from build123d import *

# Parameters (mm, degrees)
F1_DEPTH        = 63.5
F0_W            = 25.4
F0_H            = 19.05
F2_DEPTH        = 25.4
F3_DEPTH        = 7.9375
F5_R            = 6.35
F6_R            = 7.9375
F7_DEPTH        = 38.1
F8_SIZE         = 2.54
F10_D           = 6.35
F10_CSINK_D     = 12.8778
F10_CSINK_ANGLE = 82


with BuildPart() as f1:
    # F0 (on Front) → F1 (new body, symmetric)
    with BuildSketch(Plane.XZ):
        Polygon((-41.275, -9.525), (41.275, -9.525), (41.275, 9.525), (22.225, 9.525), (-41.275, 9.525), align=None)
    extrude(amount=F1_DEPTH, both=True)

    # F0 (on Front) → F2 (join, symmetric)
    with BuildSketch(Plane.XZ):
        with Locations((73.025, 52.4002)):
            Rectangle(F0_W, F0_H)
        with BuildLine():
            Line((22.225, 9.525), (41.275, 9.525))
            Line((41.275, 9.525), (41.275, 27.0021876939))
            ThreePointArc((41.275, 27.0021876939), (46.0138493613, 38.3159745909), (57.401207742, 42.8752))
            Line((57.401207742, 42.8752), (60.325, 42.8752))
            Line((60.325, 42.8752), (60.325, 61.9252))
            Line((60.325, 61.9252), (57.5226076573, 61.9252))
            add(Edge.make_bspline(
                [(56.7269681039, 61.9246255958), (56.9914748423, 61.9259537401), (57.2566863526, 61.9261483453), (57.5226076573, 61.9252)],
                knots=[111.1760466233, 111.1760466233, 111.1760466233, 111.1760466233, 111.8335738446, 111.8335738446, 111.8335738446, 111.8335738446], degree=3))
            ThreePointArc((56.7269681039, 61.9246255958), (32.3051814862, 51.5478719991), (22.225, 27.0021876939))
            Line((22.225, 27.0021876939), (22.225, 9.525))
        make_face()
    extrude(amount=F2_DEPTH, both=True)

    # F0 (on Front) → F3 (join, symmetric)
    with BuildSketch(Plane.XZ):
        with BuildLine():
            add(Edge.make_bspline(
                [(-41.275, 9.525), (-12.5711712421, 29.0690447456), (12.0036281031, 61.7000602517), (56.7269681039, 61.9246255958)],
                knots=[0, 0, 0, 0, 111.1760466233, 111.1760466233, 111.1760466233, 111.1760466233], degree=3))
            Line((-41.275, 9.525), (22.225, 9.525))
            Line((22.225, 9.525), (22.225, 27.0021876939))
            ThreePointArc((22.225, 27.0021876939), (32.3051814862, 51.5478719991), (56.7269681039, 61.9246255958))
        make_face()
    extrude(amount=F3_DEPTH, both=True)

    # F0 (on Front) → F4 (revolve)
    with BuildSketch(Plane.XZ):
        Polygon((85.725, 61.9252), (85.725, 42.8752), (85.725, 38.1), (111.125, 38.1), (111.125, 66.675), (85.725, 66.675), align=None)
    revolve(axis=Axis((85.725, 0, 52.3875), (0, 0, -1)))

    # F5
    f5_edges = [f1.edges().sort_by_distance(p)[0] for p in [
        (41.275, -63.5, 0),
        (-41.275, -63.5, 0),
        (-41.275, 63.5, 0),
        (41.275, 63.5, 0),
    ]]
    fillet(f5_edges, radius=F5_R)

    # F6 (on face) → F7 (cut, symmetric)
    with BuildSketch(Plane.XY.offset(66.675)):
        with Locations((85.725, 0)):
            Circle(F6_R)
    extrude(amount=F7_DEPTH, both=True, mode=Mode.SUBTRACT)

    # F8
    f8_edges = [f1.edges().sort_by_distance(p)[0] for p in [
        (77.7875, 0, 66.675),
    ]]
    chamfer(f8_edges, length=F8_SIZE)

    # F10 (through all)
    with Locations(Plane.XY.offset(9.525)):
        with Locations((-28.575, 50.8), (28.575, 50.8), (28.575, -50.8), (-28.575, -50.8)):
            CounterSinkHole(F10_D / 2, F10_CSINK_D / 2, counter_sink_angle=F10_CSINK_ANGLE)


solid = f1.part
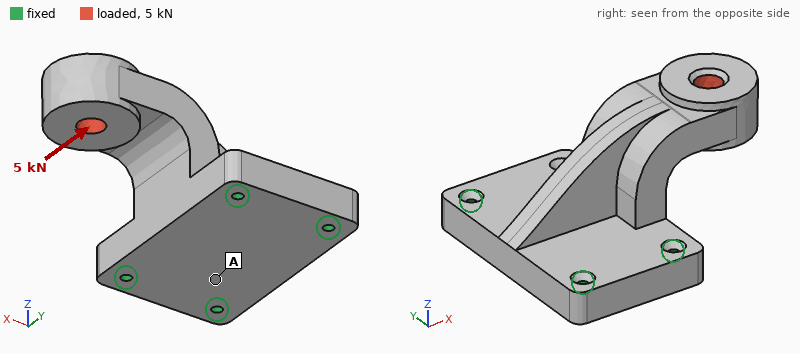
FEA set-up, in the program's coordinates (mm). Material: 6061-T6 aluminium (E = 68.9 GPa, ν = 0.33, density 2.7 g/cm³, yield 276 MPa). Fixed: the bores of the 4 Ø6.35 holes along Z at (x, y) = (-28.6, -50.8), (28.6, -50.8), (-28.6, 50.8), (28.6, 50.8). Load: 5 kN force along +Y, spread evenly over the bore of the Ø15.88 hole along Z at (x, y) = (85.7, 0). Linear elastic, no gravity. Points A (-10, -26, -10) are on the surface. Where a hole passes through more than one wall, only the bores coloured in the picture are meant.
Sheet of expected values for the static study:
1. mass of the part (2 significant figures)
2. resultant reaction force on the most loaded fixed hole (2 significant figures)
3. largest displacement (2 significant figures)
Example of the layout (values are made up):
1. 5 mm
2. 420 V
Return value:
1. 920 g
2. 4.0 kN
3. 0.27 mm
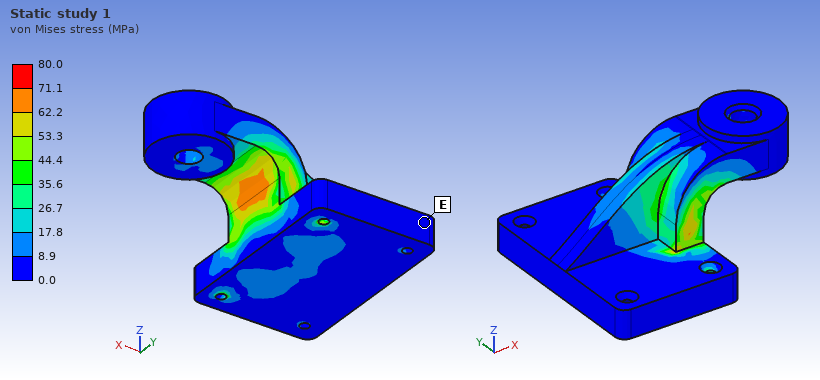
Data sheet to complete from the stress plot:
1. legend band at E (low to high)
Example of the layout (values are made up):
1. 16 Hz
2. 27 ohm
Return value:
1. 0.0 to 8.9 MPa
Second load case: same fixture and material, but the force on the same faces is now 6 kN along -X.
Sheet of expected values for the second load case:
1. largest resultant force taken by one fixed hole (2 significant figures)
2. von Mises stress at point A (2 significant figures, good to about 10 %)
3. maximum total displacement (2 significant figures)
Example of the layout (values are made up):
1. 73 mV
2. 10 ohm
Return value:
1. 3.4 kN
2. 6.5 MPa
3. 0.15 mm
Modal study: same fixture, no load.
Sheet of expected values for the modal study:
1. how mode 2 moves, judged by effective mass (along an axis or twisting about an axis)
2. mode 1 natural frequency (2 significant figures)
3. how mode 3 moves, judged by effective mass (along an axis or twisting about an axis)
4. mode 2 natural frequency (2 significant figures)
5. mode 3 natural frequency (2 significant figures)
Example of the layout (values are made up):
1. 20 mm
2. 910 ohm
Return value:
1. along Y
2. 1600 Hz
3. along X
4. 1900 Hz
5. 3900 Hz
